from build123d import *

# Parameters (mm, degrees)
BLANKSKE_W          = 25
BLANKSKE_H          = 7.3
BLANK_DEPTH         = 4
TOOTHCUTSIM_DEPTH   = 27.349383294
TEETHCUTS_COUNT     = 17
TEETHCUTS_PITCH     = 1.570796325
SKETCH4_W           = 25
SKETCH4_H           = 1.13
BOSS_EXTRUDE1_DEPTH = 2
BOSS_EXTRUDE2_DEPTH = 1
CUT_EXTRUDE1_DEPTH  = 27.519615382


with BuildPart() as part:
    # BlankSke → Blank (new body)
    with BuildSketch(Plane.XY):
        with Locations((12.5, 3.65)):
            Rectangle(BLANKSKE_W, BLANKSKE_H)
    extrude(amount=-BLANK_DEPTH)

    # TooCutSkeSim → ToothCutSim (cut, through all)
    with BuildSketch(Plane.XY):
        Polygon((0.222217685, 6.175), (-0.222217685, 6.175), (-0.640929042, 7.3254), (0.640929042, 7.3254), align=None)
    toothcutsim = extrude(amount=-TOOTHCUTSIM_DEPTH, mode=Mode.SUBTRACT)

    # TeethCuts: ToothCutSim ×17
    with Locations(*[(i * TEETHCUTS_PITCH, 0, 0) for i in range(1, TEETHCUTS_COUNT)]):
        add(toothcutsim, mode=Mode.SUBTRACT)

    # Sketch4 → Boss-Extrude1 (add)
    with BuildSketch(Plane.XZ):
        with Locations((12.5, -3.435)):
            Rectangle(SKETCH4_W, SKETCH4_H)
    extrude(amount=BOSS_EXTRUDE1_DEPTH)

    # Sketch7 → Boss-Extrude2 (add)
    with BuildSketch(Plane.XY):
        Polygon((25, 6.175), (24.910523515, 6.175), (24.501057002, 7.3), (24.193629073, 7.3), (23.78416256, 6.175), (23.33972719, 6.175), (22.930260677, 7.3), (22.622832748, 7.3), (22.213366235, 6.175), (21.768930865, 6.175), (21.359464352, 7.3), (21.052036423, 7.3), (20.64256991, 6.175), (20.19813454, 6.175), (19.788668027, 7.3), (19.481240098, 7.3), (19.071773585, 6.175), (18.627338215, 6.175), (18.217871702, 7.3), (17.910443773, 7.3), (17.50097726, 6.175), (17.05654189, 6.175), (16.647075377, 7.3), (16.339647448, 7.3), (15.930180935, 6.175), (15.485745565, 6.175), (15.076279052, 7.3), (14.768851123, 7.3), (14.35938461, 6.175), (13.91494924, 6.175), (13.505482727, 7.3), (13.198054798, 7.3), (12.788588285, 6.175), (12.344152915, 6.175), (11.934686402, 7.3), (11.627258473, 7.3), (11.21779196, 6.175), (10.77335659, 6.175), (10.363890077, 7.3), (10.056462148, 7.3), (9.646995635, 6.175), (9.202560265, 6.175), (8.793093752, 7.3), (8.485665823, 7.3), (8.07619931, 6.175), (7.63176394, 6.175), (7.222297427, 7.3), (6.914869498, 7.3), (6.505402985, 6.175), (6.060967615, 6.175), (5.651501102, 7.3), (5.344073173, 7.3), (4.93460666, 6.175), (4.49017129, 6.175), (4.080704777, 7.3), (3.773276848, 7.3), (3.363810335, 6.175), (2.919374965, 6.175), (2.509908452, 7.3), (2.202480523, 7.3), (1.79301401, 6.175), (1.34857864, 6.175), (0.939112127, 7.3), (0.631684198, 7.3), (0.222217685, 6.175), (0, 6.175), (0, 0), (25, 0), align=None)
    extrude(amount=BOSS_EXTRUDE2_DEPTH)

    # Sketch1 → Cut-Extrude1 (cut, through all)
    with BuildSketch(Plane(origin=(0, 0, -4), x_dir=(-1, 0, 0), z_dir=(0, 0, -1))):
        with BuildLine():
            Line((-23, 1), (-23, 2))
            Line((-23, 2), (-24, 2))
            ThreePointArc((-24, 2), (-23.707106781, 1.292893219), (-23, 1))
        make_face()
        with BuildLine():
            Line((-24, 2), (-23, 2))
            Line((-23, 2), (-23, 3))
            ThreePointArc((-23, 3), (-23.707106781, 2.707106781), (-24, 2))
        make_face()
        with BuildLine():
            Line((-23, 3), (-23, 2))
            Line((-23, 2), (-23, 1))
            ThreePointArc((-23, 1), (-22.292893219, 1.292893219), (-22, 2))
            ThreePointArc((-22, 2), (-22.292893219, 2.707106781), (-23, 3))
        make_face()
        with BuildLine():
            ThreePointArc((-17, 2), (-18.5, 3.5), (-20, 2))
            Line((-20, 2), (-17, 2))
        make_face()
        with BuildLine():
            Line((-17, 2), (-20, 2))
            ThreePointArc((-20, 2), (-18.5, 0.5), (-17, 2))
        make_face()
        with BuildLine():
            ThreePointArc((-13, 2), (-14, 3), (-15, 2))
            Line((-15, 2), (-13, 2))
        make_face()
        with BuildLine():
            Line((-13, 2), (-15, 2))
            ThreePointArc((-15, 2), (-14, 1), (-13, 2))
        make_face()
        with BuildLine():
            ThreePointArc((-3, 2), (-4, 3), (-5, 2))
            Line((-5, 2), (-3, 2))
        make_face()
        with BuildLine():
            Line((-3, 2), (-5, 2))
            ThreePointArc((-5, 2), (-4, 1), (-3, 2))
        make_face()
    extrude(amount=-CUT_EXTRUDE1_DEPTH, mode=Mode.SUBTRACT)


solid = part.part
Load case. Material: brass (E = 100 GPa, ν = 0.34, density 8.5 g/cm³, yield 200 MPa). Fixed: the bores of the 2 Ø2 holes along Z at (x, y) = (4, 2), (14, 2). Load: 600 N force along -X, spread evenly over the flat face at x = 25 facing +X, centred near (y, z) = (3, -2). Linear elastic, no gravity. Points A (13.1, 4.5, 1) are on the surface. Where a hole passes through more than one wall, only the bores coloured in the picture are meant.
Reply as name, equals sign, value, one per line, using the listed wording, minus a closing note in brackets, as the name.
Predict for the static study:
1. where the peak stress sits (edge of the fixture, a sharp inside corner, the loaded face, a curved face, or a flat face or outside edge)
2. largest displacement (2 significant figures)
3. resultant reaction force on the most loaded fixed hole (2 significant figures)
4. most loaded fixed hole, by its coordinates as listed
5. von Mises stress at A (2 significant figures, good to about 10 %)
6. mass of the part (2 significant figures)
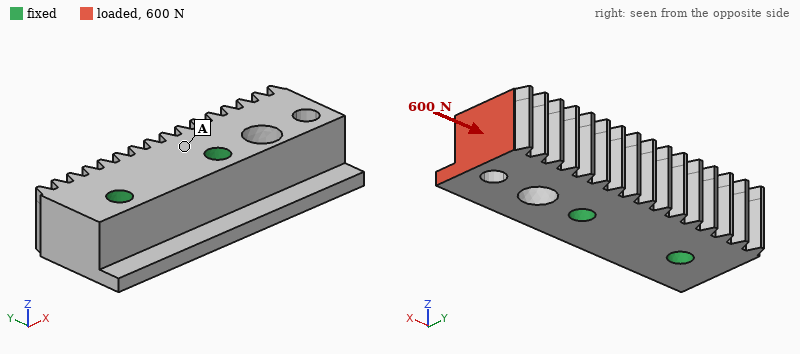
where the peak stress sits = a curved face
largest displacement = 4.4 µm
resultant reaction force on the most loaded fixed hole = 510 N
most loaded fixed hole, by its coordinates as listed = (14, 2)
von Mises stress at A = 13 MPa
mass of the part = 6.9 g
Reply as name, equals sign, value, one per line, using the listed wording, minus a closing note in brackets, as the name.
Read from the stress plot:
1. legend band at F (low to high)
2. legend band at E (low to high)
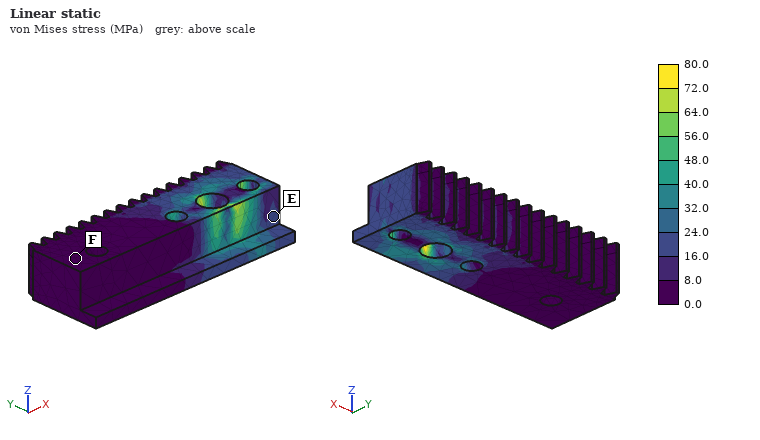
legend band at F = 0.0 to 8.0 MPa
legend band at E = 16.0 to 24.0 MPa
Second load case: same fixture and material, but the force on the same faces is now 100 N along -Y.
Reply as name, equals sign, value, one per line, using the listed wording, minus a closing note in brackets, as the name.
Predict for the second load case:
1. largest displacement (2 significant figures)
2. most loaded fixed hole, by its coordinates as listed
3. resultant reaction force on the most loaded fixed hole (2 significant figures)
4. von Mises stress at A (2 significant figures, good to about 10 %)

largest displacement = 8.7 µm
most loaded fixed hole, by its coordinates as listed = (14, 2)
resultant reaction force on the most loaded fixed hole = 170 N
von Mises stress at A = 9.7 MPa
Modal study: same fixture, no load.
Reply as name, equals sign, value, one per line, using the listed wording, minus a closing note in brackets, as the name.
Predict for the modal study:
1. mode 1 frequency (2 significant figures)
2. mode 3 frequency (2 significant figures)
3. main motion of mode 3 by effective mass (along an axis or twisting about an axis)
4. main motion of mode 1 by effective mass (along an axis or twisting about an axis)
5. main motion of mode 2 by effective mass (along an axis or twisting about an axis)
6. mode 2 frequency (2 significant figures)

mode 1 frequency = 17 kHz
mode 3 frequency = 31 kHz
main motion of mode 3 by effective mass = twisting about X
main motion of mode 1 by effective mass = along Z
main motion of mode 2 by effective mass = along Y
mode 2 frequency = 19 kHz
